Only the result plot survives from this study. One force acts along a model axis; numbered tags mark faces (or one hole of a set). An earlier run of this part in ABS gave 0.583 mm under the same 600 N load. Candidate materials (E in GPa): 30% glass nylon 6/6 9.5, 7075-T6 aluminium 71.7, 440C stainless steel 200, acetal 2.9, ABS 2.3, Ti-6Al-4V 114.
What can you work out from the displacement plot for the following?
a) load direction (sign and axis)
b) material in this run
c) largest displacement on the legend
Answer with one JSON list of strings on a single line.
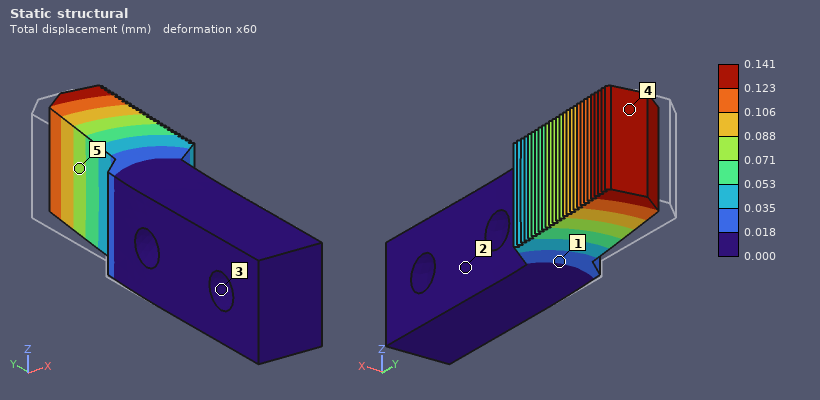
["+X", "30% glass nylon 6/6", "0.141 mm"]
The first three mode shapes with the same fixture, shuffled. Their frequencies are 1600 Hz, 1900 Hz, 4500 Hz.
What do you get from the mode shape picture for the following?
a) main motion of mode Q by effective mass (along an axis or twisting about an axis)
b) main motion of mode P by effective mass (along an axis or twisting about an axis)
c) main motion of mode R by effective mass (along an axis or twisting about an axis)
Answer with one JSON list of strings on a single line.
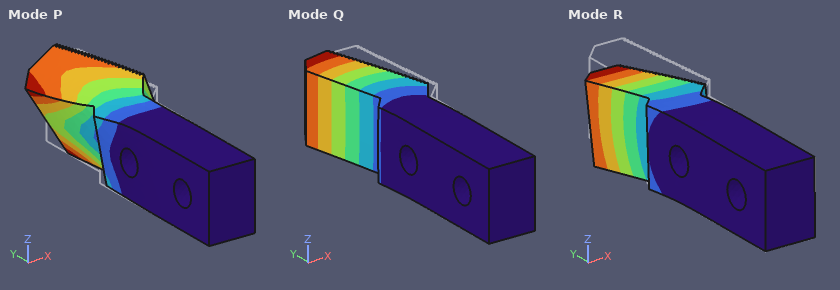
["along X", "twisting about Y", "along Z"]
